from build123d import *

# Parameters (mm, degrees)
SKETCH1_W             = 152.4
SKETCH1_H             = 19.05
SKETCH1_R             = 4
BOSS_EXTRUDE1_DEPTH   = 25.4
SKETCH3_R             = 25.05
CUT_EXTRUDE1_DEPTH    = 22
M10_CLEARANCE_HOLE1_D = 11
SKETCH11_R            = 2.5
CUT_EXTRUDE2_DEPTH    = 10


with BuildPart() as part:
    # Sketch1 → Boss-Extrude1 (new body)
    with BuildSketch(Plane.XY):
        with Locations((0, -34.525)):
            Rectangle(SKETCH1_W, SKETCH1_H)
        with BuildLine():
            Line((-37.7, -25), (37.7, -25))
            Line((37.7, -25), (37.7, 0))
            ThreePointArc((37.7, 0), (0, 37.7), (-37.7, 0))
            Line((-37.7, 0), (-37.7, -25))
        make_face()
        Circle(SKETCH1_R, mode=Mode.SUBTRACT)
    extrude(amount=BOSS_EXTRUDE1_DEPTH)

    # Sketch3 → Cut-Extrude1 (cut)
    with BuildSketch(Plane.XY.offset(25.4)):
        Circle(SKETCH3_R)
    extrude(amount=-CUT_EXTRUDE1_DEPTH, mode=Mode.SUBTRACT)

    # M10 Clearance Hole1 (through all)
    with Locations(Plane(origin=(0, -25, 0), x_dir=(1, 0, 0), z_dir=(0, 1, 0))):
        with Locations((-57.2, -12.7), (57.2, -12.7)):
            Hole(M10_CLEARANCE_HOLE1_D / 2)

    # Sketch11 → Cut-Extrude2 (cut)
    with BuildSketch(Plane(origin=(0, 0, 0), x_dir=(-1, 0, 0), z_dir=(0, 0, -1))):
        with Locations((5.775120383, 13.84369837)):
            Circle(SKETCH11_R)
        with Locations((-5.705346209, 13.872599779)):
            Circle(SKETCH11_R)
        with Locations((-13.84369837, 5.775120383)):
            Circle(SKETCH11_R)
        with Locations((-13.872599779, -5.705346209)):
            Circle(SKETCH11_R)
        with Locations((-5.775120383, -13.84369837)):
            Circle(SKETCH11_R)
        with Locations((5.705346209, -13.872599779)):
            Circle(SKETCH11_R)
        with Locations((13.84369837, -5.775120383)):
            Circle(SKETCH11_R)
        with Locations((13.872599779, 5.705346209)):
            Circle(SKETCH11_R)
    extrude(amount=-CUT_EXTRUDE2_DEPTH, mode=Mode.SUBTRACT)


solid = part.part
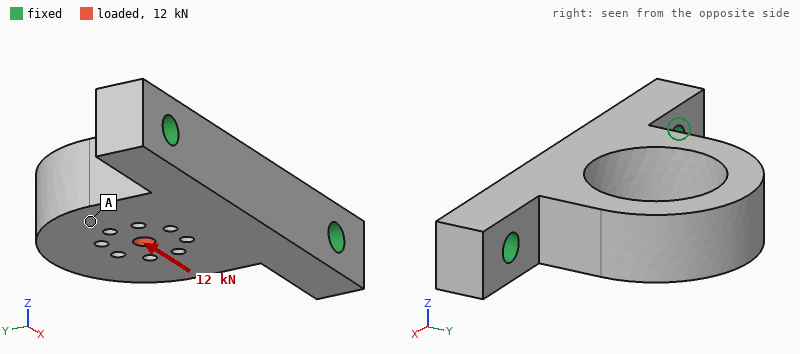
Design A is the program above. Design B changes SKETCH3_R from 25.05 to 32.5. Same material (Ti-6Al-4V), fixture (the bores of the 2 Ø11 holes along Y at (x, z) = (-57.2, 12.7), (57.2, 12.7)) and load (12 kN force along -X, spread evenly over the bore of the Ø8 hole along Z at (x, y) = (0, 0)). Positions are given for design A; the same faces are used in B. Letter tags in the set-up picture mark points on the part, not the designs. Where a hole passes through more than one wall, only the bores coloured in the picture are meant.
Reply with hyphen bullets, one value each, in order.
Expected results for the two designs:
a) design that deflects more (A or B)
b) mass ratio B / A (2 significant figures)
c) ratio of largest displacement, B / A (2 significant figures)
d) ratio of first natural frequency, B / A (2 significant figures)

- B
- 0.77
- 1.6
- 1.1
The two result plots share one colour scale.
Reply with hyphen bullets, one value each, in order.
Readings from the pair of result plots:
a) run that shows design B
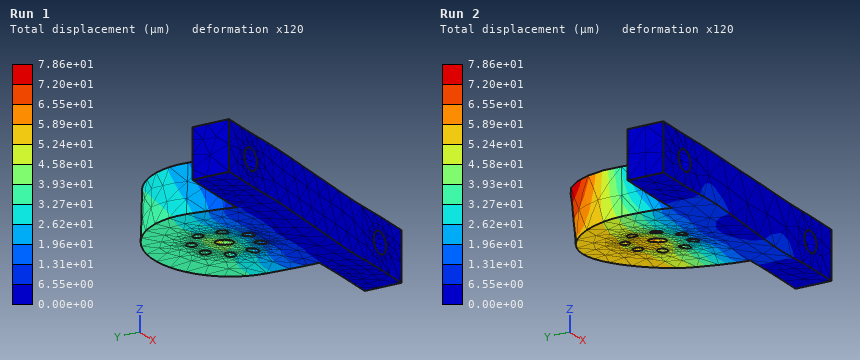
- Run 2
